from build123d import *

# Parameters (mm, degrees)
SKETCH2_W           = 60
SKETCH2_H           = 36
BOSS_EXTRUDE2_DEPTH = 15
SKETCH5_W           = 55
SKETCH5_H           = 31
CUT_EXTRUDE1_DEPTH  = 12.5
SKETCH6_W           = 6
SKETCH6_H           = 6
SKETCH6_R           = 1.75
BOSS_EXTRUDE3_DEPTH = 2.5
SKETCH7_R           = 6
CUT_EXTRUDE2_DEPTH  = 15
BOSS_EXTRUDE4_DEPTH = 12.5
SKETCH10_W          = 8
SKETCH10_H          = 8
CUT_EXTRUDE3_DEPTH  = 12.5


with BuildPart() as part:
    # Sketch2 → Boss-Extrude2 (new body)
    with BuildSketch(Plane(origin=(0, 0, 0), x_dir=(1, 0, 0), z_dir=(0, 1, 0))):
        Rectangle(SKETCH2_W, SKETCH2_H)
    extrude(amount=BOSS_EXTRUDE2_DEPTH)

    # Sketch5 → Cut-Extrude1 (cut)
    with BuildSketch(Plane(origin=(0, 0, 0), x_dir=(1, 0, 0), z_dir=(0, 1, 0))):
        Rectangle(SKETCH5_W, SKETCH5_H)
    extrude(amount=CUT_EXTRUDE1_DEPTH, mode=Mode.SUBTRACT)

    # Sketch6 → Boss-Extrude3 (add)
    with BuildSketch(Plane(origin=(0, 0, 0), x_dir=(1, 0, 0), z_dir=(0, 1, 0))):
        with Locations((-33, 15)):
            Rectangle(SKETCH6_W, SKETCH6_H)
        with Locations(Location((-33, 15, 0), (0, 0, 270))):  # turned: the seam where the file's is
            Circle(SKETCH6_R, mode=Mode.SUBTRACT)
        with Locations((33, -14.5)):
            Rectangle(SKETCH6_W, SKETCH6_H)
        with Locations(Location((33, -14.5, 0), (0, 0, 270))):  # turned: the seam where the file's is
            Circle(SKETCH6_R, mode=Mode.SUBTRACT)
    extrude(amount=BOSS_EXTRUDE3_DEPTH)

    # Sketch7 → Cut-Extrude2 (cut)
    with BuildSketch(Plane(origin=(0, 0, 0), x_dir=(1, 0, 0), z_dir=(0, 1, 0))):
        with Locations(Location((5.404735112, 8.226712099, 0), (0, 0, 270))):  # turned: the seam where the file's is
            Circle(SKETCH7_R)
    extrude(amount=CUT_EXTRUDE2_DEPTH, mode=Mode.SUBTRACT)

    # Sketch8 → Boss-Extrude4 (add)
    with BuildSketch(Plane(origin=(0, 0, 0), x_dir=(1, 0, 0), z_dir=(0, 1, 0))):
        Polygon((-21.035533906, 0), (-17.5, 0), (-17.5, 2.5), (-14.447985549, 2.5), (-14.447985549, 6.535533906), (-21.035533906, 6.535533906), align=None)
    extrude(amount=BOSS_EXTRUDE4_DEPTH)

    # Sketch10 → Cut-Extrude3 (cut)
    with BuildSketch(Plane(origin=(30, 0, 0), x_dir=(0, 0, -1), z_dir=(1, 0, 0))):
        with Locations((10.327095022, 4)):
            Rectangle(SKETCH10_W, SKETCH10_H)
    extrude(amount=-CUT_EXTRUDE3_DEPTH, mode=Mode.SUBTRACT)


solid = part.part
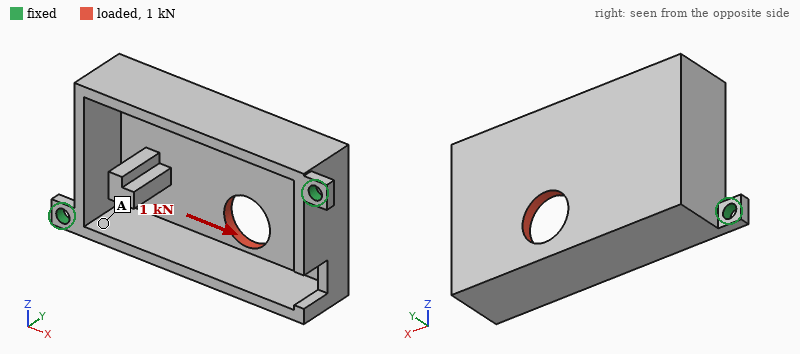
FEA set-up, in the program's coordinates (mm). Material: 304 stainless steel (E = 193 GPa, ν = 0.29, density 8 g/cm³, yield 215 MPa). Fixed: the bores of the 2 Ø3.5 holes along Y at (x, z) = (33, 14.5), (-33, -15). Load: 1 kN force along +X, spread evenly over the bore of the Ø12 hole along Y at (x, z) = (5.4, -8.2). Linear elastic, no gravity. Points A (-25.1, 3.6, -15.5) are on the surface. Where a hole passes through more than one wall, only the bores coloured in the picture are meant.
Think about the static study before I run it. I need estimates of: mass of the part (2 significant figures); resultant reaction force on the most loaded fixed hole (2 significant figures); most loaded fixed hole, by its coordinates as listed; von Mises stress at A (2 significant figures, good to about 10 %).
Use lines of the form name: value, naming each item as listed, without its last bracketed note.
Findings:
mass of the part: 90 g
resultant reaction force on the most loaded fixed hole: 650 N
most loaded fixed hole, by its coordinates as listed: (-33, -15)
von Mises stress at A: 39 MPa
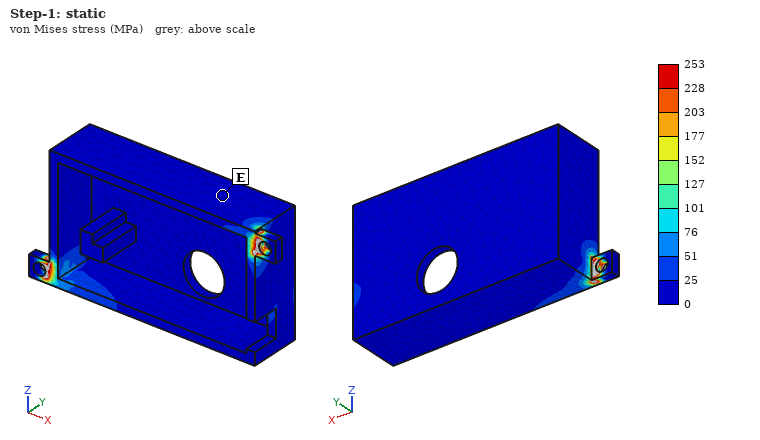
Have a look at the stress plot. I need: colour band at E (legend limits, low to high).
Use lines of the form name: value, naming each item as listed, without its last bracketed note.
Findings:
colour band at E: 0 to 25 MPa
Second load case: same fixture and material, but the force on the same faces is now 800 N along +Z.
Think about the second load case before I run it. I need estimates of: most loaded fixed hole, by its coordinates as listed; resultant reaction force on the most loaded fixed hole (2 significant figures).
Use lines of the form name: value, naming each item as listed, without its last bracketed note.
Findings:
most loaded fixed hole, by its coordinates as listed: (33, 14.5)
resultant reaction force on the most loaded fixed hole: 450 N
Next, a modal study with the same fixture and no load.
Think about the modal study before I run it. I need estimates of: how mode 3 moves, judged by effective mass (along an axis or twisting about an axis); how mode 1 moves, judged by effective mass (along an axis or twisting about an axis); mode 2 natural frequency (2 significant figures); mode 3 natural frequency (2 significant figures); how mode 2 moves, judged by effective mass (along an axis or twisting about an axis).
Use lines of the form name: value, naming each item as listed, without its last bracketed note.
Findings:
how mode 3 moves, judged by effective mass: along Z
how mode 1 moves, judged by effective mass: along Z
mode 2 natural frequency: 4700 Hz
mode 3 natural frequency: 5500 Hz
how mode 2 moves, judged by effective mass: along Y
